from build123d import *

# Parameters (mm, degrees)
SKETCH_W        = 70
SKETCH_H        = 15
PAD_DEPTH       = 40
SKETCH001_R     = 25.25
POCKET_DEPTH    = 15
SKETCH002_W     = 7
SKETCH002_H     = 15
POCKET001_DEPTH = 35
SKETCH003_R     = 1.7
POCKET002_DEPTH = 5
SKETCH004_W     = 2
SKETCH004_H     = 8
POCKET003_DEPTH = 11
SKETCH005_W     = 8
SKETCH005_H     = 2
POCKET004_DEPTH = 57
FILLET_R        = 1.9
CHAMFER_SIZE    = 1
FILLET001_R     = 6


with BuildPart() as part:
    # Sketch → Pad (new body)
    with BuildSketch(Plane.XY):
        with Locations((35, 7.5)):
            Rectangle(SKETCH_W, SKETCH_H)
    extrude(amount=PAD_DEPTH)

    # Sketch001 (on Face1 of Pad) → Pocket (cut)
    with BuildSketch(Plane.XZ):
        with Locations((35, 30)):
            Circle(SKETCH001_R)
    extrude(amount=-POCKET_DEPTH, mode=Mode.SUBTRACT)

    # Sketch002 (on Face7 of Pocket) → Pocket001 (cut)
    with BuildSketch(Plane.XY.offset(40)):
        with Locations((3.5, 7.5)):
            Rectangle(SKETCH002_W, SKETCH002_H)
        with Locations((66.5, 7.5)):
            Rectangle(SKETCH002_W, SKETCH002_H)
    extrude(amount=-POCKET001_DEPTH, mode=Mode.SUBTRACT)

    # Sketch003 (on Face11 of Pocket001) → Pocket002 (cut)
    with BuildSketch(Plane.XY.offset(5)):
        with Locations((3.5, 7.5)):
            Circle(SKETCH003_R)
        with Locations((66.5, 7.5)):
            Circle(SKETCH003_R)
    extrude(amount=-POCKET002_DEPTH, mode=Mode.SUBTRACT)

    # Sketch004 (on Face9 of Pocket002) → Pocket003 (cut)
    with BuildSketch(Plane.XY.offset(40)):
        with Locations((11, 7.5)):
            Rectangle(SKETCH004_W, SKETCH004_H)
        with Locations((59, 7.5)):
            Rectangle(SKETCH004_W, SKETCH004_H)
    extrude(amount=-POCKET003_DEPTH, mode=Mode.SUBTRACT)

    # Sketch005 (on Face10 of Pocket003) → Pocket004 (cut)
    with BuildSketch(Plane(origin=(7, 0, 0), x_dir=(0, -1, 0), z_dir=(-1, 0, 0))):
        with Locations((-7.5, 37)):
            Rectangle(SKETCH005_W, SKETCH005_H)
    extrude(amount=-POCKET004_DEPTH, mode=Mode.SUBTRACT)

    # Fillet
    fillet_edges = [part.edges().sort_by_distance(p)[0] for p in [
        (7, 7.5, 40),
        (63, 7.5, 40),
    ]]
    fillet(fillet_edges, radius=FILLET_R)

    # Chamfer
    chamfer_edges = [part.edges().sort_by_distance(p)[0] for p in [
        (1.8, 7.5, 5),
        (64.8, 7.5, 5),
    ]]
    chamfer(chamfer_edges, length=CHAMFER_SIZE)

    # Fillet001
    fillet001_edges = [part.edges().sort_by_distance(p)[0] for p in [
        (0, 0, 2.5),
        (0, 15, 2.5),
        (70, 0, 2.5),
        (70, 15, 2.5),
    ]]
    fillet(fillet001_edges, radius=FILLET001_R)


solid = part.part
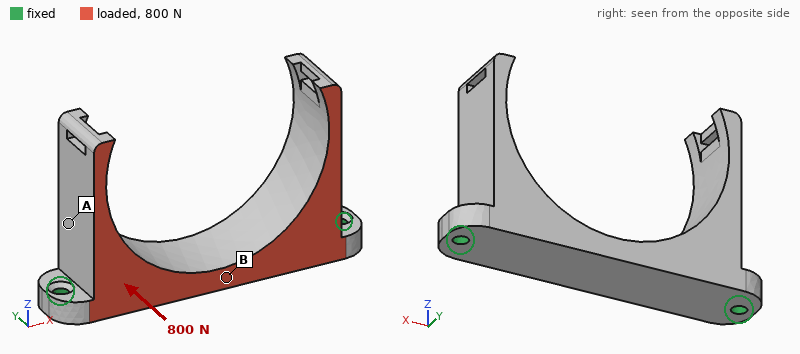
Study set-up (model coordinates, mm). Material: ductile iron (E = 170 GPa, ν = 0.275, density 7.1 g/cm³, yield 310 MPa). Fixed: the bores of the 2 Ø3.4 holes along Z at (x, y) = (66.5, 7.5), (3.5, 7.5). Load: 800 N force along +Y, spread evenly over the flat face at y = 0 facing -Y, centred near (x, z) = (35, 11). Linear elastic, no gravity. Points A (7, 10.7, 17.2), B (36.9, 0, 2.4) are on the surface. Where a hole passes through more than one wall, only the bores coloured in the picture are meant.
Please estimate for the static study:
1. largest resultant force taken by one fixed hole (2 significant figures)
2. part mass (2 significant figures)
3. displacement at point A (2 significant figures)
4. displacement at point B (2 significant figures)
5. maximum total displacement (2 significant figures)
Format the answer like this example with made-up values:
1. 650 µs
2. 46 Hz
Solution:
1. 400 N
2. 84 g
3. 11 µm
4. 6.4 µm
5. 29 µm
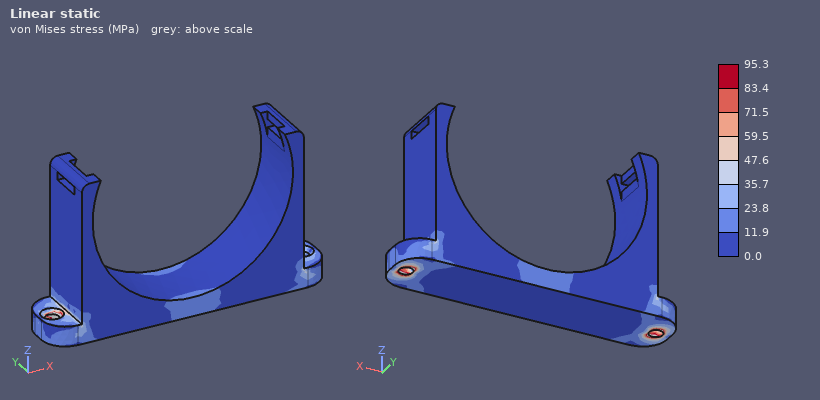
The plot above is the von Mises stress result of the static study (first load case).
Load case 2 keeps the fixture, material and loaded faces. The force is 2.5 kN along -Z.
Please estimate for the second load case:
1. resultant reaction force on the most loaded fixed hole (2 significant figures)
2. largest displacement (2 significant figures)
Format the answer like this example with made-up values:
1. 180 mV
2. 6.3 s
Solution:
1. 1.3 kN
2. 0.10 mm
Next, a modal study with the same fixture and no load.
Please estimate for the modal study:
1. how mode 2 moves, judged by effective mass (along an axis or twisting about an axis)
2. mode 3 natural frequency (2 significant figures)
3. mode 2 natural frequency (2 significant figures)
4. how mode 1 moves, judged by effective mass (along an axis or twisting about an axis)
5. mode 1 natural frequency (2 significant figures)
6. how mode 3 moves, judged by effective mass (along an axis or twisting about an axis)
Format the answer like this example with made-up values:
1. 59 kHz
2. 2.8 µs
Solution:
1. along Y
2. 5200 Hz
3. 4100 Hz
4. along Z
5. 3300 Hz
6. twisting about Z
